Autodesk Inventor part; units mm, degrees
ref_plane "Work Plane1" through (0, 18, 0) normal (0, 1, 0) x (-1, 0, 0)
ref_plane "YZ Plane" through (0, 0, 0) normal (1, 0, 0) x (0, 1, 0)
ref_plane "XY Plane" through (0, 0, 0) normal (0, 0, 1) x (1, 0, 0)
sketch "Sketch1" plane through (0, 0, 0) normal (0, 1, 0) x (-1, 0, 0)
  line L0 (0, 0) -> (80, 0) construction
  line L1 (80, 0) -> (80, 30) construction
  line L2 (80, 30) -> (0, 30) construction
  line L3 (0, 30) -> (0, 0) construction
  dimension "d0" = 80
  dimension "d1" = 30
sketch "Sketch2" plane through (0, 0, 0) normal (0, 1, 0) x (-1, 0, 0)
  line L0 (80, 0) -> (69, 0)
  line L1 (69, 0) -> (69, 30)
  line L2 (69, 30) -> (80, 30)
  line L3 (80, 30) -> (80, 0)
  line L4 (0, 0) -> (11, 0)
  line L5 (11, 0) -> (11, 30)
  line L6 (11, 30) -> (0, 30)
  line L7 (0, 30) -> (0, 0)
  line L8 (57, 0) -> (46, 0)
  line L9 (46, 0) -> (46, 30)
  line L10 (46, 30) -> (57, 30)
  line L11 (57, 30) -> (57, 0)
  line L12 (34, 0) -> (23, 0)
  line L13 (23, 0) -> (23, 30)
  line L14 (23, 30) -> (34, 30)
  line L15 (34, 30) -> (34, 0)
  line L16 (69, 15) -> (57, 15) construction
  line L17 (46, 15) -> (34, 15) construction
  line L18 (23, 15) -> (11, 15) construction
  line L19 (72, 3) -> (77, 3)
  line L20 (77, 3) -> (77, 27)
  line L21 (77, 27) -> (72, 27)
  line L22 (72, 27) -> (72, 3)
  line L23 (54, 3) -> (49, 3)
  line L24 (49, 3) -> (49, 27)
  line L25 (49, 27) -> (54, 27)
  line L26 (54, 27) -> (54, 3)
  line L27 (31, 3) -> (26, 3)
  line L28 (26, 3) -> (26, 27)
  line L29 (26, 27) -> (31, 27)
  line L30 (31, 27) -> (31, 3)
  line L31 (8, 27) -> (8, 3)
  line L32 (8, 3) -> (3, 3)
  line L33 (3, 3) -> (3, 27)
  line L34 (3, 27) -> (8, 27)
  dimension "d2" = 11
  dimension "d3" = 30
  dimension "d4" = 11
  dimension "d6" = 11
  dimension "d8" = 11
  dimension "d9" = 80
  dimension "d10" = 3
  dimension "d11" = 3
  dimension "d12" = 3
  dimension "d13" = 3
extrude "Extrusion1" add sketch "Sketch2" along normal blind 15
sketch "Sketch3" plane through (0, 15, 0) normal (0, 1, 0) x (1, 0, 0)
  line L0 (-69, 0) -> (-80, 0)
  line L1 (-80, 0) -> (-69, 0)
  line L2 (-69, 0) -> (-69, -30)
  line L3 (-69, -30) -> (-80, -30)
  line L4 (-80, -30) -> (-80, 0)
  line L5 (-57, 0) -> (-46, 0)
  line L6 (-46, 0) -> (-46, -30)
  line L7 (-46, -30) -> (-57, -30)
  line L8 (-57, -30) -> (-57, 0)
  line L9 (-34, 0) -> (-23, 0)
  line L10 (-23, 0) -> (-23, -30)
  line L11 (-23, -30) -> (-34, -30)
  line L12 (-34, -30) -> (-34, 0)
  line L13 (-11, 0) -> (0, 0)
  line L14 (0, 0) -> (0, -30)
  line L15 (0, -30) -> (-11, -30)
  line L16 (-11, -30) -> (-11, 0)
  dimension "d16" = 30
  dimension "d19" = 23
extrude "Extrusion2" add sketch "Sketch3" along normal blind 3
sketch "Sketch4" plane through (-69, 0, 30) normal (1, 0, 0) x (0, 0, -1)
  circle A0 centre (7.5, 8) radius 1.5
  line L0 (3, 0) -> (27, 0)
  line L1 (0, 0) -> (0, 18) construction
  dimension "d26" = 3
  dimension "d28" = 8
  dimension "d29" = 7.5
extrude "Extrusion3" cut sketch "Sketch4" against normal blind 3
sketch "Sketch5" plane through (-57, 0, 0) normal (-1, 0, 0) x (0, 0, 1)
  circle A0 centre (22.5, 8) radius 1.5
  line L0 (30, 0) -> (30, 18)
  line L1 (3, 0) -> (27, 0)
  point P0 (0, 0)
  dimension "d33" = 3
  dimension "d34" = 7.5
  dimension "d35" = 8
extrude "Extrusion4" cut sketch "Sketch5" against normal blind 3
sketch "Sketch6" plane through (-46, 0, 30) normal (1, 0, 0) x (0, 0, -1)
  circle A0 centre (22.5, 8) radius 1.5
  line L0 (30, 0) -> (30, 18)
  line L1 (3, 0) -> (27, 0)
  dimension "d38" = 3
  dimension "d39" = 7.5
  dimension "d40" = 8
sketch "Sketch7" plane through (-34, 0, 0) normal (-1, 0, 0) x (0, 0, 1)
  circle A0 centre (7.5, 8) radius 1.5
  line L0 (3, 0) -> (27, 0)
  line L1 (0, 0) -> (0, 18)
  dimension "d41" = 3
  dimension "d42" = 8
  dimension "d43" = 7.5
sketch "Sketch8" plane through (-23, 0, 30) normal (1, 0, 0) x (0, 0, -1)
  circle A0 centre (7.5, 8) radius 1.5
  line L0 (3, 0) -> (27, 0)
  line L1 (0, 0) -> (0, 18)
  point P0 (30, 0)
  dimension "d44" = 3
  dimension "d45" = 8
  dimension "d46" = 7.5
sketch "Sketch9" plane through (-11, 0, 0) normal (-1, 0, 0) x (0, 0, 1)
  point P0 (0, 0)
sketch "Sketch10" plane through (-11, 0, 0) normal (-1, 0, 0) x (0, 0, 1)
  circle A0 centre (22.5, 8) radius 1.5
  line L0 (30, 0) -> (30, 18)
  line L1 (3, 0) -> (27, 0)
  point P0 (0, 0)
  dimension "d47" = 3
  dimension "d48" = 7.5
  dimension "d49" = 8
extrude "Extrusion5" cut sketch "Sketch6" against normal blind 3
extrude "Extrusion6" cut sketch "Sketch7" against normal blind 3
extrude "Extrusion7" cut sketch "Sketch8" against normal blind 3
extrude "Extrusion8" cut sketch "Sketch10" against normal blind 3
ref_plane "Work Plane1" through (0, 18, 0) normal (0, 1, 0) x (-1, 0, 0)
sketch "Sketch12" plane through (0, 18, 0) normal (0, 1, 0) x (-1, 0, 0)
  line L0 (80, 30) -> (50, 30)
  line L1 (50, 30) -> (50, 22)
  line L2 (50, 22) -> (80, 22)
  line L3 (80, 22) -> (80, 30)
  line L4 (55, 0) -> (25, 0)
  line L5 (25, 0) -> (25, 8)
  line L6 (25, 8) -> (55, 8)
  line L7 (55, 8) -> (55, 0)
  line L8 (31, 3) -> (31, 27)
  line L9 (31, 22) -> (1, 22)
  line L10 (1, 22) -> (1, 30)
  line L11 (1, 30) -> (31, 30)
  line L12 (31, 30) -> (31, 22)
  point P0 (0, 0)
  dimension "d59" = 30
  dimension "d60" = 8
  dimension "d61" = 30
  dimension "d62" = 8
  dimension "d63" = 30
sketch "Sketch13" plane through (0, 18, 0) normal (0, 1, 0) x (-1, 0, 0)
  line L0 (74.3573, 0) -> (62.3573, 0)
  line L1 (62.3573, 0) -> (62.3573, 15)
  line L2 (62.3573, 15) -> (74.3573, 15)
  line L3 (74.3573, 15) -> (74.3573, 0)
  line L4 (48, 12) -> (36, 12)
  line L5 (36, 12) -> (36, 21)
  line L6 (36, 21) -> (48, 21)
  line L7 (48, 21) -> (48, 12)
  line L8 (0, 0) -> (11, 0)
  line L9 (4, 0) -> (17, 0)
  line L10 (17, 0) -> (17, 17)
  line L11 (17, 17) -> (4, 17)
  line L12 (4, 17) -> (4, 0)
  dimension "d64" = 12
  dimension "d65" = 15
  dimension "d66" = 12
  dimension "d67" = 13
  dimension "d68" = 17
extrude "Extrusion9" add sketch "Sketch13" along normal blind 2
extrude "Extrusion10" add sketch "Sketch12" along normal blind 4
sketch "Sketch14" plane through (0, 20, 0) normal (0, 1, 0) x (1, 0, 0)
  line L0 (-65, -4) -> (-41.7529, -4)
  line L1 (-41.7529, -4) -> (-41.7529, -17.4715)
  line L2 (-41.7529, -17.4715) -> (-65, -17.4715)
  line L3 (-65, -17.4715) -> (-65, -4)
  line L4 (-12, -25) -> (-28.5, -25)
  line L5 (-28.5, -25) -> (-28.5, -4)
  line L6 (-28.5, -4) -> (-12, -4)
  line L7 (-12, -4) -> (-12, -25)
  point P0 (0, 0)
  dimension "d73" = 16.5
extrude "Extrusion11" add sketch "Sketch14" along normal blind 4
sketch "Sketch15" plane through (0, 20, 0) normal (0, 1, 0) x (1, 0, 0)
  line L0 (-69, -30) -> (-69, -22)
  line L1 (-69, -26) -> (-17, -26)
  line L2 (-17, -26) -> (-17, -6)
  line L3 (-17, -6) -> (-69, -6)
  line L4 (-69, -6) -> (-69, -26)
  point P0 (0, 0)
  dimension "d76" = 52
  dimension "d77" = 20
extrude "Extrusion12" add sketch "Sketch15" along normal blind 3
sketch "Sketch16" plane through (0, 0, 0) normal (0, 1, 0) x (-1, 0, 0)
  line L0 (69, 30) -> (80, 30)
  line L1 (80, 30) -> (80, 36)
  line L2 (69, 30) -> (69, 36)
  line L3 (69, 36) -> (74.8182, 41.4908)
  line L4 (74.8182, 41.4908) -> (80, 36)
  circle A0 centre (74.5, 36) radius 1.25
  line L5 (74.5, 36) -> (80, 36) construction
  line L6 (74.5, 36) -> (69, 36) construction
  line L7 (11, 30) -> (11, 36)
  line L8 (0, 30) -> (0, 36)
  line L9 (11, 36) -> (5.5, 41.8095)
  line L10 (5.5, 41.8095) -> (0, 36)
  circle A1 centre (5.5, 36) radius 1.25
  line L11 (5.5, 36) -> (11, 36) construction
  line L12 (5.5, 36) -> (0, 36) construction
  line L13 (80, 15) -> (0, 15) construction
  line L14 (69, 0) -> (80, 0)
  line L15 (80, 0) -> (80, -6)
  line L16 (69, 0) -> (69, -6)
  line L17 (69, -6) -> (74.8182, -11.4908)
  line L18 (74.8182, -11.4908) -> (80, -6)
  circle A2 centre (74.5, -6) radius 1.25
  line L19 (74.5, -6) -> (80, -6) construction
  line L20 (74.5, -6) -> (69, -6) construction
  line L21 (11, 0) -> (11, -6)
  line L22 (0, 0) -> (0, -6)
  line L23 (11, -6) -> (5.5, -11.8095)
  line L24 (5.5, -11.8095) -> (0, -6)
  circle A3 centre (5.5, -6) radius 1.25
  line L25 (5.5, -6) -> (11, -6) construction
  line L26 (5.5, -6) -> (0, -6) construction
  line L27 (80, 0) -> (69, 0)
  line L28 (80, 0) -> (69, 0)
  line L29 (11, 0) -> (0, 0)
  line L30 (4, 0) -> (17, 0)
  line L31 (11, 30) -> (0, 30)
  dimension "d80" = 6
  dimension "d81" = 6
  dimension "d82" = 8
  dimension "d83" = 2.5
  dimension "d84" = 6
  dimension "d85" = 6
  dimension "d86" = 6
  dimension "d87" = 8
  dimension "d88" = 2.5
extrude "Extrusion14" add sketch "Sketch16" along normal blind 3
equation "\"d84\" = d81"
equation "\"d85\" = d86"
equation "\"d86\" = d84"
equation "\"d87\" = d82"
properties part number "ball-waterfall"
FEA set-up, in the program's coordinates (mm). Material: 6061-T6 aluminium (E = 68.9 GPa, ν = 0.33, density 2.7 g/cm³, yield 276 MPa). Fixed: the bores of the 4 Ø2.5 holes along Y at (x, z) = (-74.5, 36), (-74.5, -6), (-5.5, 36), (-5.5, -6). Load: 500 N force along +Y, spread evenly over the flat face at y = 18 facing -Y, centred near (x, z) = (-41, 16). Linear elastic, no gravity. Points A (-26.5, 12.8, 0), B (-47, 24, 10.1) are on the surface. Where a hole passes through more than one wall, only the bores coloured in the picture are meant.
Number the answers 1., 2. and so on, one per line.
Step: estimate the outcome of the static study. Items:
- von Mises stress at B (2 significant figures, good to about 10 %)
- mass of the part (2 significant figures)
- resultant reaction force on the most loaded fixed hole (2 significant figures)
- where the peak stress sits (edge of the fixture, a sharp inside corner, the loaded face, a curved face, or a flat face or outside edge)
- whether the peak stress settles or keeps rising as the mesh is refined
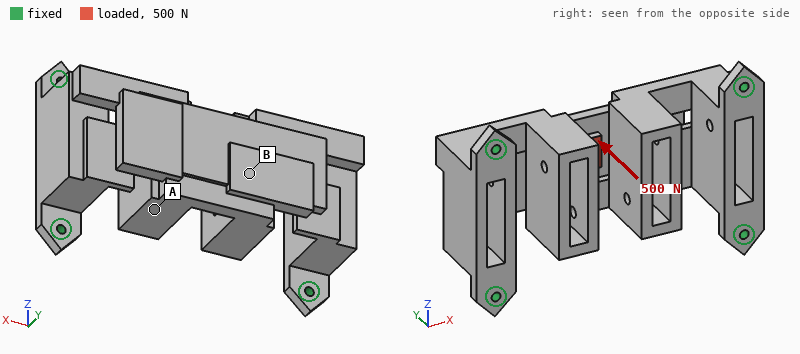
1. 25 MPa
2. 68 g
3. 200 N
4. edge of the fixture
5. keeps rising
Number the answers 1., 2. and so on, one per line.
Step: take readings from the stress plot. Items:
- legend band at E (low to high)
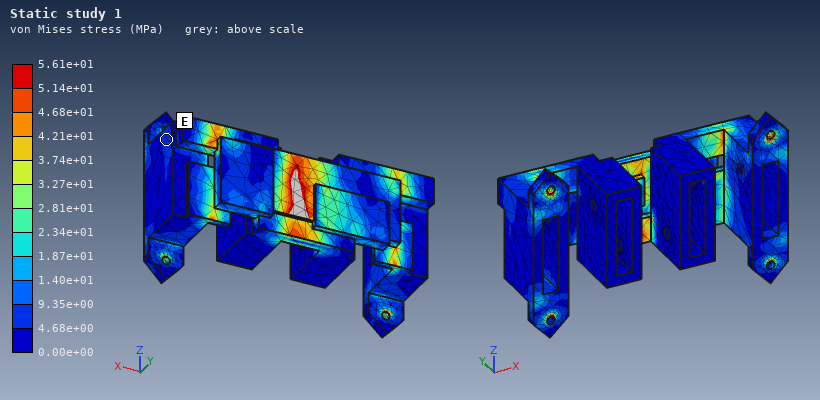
1. 4.68e+00 to 9.35e+00 MPa
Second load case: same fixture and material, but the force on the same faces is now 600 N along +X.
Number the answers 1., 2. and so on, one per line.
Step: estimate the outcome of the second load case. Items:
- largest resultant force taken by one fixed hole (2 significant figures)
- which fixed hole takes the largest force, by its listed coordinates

1. 180 N
2. (-74.5, 36)
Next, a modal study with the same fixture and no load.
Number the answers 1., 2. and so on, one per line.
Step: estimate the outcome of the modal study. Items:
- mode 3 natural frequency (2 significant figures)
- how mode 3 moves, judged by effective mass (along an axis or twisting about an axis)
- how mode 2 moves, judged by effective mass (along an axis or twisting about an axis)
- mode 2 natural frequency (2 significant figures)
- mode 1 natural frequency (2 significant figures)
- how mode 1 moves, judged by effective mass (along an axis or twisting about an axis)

1. 3400 Hz
2. along Z
3. along Y
4. 2400 Hz
5. 1900 Hz
6. along X
